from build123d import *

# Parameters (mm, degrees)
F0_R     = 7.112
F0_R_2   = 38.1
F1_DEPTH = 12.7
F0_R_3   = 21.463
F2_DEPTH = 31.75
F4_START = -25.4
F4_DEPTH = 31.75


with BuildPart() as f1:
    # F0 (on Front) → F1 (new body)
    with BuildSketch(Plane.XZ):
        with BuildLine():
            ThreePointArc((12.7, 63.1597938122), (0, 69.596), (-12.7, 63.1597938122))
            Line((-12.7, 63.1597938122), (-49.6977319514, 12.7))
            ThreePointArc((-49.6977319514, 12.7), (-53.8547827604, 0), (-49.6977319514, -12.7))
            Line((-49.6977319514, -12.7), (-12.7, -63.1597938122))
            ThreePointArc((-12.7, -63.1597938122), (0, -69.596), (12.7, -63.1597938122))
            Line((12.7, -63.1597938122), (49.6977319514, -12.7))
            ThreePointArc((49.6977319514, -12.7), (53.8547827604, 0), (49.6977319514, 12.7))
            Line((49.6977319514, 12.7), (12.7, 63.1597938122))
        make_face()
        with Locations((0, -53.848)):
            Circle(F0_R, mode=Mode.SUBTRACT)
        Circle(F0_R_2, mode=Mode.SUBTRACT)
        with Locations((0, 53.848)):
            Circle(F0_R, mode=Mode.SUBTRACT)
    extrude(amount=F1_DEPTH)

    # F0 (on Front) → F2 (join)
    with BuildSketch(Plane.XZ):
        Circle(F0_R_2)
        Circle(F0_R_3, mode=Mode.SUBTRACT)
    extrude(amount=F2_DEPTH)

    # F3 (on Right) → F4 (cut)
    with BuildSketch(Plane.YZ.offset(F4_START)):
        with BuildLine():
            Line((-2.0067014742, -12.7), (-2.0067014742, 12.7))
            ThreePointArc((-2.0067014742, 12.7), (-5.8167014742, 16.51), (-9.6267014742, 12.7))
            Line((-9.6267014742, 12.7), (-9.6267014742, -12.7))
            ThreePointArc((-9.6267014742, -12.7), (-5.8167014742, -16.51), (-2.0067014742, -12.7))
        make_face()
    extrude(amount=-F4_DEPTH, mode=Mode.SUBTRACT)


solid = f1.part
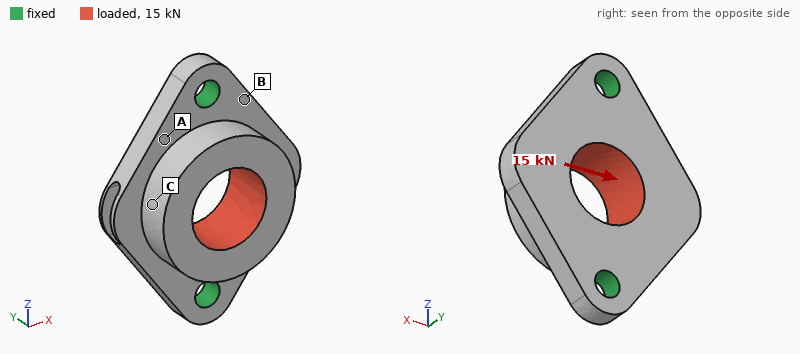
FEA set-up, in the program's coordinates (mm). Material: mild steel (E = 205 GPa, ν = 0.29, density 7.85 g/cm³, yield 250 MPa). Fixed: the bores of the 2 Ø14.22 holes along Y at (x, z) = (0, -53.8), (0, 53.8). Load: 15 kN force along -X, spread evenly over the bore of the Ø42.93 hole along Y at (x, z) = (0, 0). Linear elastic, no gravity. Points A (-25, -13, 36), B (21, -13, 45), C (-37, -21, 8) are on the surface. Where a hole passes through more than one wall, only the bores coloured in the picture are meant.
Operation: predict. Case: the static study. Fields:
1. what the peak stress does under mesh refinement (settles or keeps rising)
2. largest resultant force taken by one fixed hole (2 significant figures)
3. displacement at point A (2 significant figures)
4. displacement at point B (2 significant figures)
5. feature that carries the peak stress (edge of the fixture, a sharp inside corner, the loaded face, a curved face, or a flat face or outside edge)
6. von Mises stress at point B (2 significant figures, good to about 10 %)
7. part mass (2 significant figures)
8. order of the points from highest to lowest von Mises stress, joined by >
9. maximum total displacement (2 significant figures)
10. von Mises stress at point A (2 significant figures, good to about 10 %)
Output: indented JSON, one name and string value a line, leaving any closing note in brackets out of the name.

{
  "what the peak stress does under mesh refinement": "keeps rising",
  "largest resultant force taken by one fixed hole": "7.5 kN",
  "displacement at point A": "12 µm",
  "displacement at point B": "7.5 µm",
  "feature that carries the peak stress": "edge of the fixture",
  "von Mises stress at point B": "29 MPa",
  "part mass": "1.2 kg",
  "order of the points from highest to lowest von Mises stress, joined by >": "B > A > C",
  "maximum total displacement": "29 µm",
  "von Mises stress at point A": "17 MPa"
}
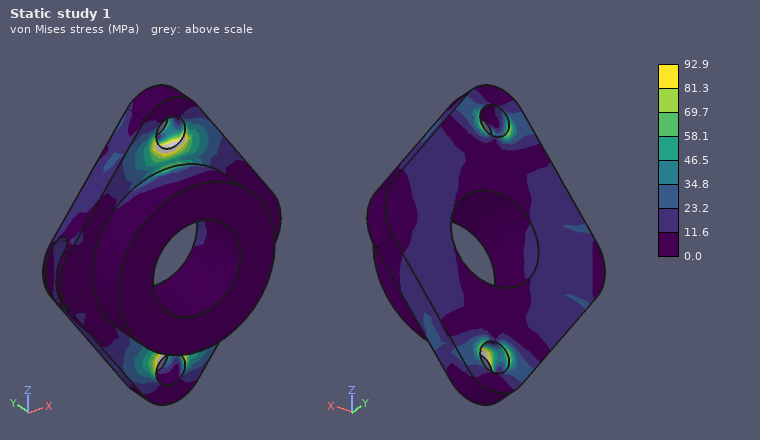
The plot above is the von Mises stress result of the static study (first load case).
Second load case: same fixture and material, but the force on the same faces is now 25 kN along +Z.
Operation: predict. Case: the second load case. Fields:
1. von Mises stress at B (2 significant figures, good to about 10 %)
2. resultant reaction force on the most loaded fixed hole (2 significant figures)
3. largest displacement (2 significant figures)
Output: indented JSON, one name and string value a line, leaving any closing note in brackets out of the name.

{
  "von Mises stress at B": "15 MPa",
  "resultant reaction force on the most loaded fixed hole": "13 kN",
  "largest displacement": "6.2 µm"
}
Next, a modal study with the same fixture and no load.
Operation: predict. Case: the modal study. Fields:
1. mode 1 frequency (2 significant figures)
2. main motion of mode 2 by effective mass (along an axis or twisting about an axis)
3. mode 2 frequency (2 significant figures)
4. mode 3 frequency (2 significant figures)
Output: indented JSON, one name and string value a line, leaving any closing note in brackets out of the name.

{
  "mode 1 frequency": "3100 Hz",
  "main motion of mode 2 by effective mass": "along Y",
  "mode 2 frequency": "5100 Hz",
  "mode 3 frequency": "8900 Hz"
}
